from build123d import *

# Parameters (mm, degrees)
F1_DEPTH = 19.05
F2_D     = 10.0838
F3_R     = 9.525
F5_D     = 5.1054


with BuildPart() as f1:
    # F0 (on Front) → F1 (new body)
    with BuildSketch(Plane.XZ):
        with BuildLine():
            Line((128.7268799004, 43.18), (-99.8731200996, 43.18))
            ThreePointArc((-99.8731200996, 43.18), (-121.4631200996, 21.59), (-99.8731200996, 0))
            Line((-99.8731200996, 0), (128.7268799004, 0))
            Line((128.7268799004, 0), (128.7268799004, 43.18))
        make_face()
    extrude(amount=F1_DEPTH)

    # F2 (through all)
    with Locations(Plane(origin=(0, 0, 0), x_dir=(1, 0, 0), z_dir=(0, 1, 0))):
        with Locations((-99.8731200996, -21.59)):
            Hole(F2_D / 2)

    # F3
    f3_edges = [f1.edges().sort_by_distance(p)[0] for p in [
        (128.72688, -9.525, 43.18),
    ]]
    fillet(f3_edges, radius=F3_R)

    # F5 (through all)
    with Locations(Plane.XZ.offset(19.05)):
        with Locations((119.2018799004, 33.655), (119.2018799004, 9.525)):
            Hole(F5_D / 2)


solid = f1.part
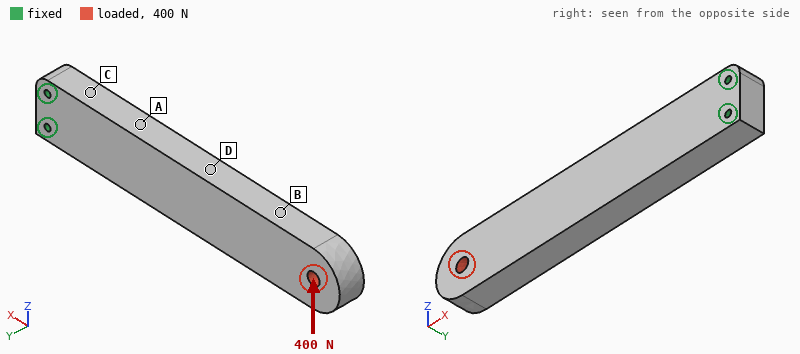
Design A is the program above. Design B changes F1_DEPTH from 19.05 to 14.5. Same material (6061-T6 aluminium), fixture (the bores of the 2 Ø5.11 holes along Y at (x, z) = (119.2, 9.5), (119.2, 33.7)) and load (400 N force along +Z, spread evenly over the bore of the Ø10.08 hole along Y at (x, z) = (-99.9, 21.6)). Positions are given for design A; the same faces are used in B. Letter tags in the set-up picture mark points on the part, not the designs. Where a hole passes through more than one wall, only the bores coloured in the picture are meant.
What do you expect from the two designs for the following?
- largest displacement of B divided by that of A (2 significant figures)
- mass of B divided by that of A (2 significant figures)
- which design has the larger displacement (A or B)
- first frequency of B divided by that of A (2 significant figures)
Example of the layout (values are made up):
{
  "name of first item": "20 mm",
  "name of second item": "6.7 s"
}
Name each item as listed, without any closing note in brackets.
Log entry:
{
  "largest displacement of B divided by that of A": "1.3",
  "mass of B divided by that of A": "0.76",
  "which design has the larger displacement": "B",
  "first frequency of B divided by that of A": "0.77"
}
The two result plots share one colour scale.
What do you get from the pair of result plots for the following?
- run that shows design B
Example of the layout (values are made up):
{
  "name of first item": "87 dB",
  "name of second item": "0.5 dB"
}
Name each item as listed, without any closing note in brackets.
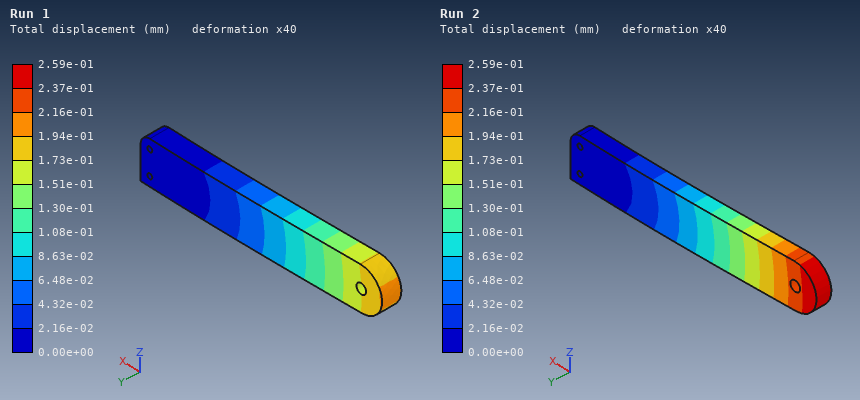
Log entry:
{
  "run that shows design B": "Run 2"
}
